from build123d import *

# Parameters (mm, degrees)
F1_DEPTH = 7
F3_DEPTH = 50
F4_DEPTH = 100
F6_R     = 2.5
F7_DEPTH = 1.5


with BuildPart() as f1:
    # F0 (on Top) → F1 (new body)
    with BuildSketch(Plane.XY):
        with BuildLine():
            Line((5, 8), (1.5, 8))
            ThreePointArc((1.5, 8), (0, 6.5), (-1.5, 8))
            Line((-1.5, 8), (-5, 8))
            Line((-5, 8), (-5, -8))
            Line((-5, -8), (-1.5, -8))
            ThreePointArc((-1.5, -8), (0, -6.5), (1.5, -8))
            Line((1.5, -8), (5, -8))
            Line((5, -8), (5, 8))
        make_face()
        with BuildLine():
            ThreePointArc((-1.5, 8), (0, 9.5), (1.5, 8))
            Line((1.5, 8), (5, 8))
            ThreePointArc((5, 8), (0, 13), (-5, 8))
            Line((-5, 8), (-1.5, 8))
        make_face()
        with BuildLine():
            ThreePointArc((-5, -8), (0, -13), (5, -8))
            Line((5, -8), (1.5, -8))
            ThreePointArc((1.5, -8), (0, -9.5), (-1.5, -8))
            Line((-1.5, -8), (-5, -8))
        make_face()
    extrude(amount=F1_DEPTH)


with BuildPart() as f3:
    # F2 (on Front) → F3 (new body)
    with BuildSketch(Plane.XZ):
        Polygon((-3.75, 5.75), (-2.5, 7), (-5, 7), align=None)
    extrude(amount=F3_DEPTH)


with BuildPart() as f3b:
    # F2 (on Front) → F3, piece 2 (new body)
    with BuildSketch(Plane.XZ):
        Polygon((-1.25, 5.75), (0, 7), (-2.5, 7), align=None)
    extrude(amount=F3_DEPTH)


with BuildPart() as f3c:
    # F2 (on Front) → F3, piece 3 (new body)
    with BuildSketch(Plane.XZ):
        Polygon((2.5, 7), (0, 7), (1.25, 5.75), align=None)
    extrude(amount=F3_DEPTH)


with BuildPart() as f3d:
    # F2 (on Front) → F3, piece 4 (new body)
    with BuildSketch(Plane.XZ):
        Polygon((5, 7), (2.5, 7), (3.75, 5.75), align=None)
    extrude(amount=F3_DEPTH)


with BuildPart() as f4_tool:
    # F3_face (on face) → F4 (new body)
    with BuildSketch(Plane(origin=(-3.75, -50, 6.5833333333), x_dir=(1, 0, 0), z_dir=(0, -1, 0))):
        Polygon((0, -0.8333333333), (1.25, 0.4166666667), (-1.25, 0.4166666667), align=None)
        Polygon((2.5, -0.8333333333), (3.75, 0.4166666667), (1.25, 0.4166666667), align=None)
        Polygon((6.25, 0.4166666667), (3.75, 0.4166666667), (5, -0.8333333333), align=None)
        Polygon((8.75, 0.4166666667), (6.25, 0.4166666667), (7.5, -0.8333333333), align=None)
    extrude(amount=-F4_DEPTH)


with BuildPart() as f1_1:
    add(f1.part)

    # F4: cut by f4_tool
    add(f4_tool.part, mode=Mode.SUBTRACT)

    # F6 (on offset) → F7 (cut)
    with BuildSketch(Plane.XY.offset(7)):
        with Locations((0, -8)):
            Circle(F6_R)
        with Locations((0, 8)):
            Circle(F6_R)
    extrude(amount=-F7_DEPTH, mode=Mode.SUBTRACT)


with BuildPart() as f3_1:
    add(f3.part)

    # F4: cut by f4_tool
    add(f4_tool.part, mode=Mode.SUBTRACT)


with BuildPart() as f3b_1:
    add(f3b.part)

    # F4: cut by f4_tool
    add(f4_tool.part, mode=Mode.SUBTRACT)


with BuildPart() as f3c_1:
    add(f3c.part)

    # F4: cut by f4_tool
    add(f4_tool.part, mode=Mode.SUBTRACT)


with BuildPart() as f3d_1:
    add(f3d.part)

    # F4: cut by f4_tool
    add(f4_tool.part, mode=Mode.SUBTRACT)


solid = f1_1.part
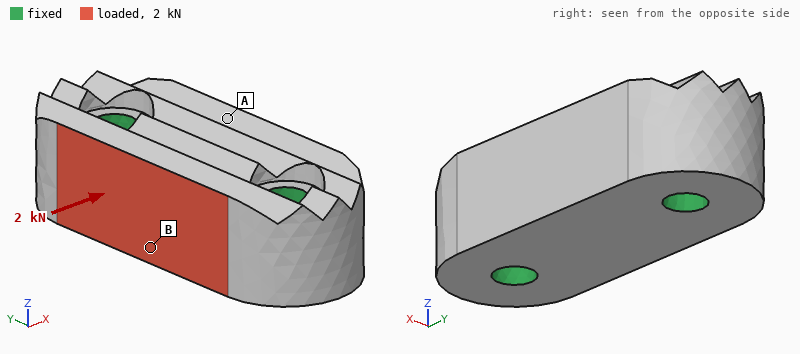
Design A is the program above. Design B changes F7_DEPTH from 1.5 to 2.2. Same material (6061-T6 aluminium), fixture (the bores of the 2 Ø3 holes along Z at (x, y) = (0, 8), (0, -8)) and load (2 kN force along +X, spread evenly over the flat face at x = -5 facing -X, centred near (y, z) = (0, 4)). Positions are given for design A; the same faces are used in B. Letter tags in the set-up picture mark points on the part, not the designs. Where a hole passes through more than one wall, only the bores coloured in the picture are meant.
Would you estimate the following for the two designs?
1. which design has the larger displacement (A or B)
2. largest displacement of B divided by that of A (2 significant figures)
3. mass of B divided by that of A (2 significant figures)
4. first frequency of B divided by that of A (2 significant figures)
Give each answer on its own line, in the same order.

B
1.2
0.99
0.88
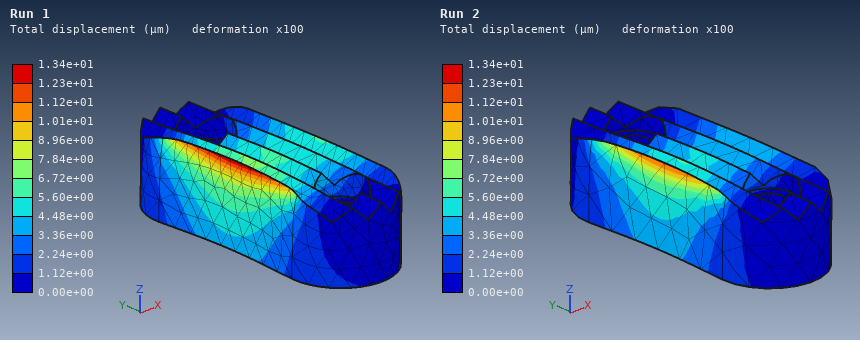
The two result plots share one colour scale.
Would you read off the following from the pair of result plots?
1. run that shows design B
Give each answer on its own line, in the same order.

Run 1
